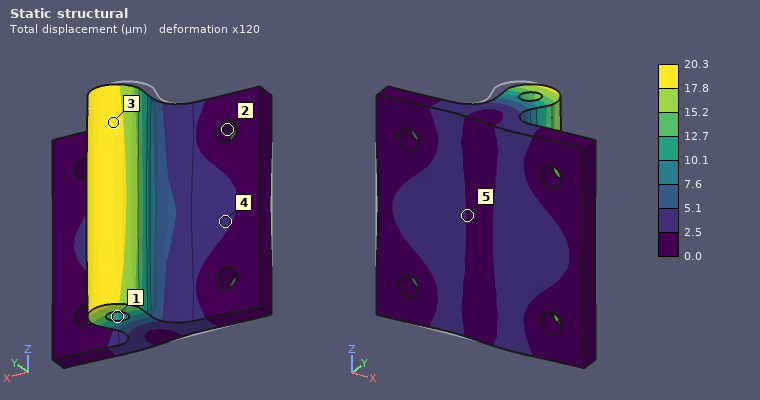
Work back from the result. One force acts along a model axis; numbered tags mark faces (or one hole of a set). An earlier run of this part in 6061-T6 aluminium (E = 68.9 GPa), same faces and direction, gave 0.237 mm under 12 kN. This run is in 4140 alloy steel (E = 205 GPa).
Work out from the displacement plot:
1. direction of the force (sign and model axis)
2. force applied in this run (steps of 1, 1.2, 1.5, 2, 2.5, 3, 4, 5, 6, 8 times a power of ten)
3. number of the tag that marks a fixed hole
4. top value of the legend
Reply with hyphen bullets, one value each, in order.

- +X
- 3 kN
- 2
- 20.3 µm
